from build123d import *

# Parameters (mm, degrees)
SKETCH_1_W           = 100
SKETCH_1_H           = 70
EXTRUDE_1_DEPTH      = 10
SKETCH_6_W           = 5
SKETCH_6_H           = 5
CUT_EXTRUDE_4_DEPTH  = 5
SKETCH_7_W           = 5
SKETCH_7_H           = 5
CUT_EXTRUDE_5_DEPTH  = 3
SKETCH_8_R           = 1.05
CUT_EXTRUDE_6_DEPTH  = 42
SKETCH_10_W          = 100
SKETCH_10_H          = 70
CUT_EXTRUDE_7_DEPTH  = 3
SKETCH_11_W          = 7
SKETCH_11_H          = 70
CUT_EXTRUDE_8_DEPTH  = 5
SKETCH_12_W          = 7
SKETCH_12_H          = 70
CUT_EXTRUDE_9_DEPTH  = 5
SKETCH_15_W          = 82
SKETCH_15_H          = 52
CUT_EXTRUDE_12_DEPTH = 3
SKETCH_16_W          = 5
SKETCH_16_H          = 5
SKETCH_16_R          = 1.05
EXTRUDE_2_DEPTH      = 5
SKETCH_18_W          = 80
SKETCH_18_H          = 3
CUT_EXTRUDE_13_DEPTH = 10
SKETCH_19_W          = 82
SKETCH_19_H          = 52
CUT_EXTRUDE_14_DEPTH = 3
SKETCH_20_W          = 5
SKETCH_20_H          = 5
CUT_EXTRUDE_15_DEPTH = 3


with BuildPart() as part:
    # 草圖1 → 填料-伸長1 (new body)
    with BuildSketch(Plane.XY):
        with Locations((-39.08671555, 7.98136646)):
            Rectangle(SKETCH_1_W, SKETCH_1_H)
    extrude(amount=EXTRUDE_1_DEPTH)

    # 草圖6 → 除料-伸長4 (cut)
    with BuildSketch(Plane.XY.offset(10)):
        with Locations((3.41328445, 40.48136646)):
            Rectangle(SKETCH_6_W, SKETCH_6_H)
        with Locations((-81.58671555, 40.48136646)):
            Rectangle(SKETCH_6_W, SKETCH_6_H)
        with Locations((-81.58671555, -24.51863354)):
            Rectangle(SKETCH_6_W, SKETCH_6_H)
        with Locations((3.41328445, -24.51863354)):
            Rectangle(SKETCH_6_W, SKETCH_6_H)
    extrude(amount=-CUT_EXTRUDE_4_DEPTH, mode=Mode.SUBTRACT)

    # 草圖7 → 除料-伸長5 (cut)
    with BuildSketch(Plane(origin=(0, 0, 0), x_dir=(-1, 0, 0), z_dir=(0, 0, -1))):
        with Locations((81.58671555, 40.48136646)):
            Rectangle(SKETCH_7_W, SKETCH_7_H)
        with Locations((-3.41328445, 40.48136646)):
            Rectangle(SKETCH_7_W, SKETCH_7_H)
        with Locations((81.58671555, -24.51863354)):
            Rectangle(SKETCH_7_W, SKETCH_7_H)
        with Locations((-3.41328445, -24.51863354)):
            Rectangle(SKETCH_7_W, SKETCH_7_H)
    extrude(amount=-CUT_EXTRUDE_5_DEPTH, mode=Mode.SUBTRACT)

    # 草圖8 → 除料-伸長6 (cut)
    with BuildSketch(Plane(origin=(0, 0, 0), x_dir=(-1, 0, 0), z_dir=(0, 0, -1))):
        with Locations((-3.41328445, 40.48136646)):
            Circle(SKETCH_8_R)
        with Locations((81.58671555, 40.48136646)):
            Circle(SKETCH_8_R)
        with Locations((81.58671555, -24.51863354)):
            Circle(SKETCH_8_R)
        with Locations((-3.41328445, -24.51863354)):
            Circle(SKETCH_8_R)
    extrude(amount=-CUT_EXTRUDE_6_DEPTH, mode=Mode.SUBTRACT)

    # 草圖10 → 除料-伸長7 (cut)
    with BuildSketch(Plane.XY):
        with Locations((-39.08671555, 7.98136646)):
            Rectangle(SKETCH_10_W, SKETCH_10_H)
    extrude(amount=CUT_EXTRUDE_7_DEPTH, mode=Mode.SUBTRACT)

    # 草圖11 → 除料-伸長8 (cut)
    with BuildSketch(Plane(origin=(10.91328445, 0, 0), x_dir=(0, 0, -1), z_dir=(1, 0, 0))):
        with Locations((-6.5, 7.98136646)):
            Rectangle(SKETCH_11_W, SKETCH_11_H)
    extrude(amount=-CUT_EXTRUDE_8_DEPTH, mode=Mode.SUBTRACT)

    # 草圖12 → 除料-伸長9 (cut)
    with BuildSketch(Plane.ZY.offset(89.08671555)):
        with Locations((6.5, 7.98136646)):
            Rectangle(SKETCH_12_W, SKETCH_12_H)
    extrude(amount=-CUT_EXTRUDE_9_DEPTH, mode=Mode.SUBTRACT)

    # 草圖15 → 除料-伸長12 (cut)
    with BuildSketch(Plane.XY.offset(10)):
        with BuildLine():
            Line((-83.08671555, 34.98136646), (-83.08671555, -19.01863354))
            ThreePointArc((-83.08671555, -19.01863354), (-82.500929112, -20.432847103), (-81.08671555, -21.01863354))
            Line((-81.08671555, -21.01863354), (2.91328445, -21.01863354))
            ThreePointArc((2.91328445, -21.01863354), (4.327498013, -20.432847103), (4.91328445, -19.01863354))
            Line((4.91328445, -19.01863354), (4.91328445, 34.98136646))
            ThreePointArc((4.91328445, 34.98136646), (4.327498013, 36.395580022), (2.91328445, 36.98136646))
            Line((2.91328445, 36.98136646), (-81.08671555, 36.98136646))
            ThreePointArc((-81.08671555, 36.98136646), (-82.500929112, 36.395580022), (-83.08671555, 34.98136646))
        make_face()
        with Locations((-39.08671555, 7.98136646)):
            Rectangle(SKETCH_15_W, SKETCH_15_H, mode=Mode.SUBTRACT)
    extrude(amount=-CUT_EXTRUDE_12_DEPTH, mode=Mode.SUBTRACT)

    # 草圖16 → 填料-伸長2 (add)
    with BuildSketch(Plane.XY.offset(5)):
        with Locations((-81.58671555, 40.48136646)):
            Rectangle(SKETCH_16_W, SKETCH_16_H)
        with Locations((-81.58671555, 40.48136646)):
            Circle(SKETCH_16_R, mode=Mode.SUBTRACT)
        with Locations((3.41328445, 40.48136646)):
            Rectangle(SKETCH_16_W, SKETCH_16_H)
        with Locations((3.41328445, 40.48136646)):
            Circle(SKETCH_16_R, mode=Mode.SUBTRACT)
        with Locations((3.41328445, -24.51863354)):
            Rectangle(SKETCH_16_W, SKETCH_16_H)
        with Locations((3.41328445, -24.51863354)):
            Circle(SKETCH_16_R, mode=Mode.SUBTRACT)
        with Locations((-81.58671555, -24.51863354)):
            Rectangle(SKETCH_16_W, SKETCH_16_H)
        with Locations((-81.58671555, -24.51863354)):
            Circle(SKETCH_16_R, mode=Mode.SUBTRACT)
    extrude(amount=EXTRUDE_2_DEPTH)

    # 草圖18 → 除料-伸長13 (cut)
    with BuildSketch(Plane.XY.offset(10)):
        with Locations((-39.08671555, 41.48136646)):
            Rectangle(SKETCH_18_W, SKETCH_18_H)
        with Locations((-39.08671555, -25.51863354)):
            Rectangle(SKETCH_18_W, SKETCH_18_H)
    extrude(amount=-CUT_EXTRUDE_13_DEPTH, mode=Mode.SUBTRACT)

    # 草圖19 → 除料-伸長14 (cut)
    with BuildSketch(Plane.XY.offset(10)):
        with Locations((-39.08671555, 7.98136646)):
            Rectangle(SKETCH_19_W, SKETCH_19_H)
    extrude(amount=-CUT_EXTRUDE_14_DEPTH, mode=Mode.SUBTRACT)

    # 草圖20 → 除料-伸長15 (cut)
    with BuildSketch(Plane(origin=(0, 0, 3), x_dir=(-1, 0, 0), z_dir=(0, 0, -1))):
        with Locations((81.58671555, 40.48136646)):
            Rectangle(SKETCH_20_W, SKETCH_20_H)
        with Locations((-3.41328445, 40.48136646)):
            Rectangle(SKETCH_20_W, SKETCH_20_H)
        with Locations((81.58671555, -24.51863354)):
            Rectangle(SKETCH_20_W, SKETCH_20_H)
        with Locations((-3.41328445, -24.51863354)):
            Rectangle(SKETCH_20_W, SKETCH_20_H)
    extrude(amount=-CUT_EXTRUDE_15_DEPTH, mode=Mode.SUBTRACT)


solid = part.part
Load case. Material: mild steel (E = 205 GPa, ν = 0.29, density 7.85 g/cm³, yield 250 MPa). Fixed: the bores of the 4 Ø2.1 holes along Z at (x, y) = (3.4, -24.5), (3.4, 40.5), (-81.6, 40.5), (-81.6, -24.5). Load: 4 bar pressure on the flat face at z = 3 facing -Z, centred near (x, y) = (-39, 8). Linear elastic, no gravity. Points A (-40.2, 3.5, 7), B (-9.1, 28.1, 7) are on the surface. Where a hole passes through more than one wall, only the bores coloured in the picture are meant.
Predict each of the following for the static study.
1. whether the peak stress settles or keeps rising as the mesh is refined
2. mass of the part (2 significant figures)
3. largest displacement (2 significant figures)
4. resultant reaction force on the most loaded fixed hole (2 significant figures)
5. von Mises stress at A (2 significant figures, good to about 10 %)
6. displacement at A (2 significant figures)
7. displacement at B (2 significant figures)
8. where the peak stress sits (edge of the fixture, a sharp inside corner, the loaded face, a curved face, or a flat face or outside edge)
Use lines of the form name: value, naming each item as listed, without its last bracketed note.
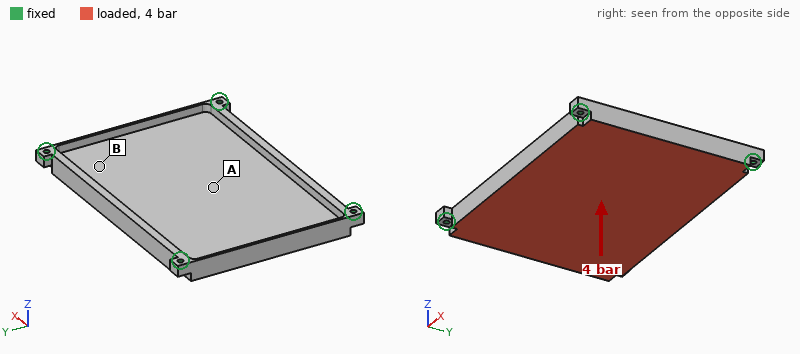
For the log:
whether the peak stress settles or keeps rising as the mesh is refined: keeps rising
mass of the part: 200 g
largest displacement: 84 µm
resultant reaction force on the most loaded fixed hole: 1.5 kN
von Mises stress at A: 38 MPa
displacement at A: 84 µm
displacement at B: 35 µm
where the peak stress sits: edge of the fixture
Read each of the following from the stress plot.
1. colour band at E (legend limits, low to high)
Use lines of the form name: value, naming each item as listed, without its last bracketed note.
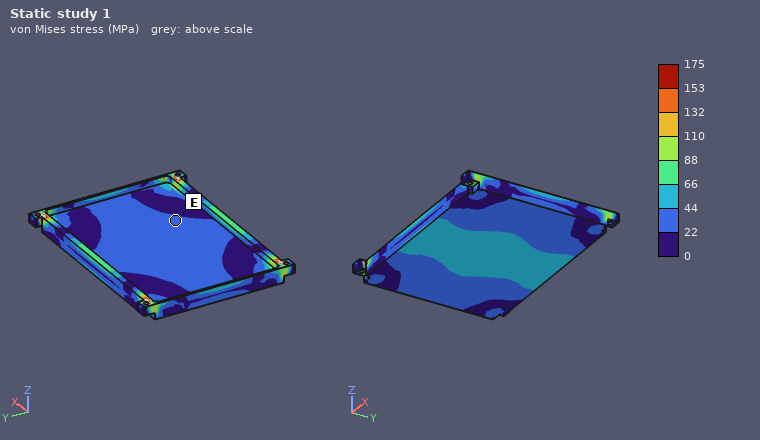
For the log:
colour band at E: 22 to 44 MPa
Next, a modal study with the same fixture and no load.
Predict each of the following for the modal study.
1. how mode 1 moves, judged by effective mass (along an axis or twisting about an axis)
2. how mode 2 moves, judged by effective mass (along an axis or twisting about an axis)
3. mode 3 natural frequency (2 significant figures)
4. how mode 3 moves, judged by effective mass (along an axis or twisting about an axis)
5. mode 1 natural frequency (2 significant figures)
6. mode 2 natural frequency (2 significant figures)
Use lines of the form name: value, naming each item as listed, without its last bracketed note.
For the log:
how mode 1 moves, judged by effective mass: along Z
how mode 2 moves, judged by effective mass: twisting about X
mode 3 natural frequency: 4600 Hz
how mode 3 moves, judged by effective mass: twisting about Y
mode 1 natural frequency: 2300 Hz
mode 2 natural frequency: 3800 Hz
